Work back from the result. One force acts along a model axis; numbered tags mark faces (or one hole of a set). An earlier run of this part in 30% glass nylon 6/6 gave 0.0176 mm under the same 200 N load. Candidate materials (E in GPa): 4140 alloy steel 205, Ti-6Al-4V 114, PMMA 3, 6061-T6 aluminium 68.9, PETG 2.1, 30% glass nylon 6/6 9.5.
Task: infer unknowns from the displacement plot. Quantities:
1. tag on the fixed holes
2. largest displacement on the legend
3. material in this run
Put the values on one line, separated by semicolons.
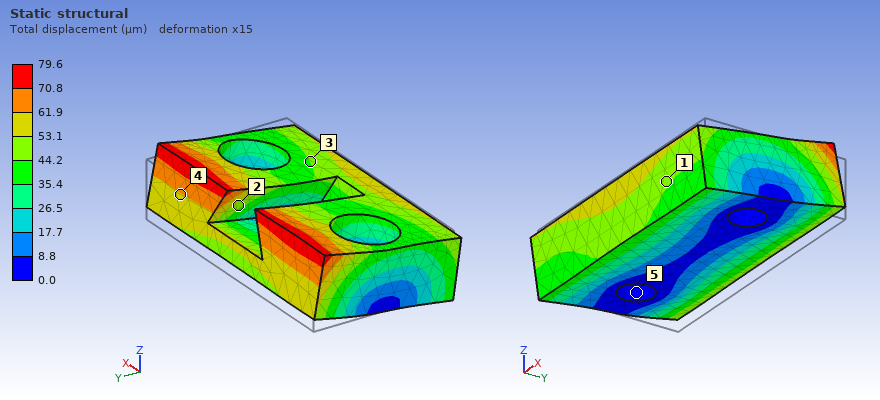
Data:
5; 79.6 µm; PETG
